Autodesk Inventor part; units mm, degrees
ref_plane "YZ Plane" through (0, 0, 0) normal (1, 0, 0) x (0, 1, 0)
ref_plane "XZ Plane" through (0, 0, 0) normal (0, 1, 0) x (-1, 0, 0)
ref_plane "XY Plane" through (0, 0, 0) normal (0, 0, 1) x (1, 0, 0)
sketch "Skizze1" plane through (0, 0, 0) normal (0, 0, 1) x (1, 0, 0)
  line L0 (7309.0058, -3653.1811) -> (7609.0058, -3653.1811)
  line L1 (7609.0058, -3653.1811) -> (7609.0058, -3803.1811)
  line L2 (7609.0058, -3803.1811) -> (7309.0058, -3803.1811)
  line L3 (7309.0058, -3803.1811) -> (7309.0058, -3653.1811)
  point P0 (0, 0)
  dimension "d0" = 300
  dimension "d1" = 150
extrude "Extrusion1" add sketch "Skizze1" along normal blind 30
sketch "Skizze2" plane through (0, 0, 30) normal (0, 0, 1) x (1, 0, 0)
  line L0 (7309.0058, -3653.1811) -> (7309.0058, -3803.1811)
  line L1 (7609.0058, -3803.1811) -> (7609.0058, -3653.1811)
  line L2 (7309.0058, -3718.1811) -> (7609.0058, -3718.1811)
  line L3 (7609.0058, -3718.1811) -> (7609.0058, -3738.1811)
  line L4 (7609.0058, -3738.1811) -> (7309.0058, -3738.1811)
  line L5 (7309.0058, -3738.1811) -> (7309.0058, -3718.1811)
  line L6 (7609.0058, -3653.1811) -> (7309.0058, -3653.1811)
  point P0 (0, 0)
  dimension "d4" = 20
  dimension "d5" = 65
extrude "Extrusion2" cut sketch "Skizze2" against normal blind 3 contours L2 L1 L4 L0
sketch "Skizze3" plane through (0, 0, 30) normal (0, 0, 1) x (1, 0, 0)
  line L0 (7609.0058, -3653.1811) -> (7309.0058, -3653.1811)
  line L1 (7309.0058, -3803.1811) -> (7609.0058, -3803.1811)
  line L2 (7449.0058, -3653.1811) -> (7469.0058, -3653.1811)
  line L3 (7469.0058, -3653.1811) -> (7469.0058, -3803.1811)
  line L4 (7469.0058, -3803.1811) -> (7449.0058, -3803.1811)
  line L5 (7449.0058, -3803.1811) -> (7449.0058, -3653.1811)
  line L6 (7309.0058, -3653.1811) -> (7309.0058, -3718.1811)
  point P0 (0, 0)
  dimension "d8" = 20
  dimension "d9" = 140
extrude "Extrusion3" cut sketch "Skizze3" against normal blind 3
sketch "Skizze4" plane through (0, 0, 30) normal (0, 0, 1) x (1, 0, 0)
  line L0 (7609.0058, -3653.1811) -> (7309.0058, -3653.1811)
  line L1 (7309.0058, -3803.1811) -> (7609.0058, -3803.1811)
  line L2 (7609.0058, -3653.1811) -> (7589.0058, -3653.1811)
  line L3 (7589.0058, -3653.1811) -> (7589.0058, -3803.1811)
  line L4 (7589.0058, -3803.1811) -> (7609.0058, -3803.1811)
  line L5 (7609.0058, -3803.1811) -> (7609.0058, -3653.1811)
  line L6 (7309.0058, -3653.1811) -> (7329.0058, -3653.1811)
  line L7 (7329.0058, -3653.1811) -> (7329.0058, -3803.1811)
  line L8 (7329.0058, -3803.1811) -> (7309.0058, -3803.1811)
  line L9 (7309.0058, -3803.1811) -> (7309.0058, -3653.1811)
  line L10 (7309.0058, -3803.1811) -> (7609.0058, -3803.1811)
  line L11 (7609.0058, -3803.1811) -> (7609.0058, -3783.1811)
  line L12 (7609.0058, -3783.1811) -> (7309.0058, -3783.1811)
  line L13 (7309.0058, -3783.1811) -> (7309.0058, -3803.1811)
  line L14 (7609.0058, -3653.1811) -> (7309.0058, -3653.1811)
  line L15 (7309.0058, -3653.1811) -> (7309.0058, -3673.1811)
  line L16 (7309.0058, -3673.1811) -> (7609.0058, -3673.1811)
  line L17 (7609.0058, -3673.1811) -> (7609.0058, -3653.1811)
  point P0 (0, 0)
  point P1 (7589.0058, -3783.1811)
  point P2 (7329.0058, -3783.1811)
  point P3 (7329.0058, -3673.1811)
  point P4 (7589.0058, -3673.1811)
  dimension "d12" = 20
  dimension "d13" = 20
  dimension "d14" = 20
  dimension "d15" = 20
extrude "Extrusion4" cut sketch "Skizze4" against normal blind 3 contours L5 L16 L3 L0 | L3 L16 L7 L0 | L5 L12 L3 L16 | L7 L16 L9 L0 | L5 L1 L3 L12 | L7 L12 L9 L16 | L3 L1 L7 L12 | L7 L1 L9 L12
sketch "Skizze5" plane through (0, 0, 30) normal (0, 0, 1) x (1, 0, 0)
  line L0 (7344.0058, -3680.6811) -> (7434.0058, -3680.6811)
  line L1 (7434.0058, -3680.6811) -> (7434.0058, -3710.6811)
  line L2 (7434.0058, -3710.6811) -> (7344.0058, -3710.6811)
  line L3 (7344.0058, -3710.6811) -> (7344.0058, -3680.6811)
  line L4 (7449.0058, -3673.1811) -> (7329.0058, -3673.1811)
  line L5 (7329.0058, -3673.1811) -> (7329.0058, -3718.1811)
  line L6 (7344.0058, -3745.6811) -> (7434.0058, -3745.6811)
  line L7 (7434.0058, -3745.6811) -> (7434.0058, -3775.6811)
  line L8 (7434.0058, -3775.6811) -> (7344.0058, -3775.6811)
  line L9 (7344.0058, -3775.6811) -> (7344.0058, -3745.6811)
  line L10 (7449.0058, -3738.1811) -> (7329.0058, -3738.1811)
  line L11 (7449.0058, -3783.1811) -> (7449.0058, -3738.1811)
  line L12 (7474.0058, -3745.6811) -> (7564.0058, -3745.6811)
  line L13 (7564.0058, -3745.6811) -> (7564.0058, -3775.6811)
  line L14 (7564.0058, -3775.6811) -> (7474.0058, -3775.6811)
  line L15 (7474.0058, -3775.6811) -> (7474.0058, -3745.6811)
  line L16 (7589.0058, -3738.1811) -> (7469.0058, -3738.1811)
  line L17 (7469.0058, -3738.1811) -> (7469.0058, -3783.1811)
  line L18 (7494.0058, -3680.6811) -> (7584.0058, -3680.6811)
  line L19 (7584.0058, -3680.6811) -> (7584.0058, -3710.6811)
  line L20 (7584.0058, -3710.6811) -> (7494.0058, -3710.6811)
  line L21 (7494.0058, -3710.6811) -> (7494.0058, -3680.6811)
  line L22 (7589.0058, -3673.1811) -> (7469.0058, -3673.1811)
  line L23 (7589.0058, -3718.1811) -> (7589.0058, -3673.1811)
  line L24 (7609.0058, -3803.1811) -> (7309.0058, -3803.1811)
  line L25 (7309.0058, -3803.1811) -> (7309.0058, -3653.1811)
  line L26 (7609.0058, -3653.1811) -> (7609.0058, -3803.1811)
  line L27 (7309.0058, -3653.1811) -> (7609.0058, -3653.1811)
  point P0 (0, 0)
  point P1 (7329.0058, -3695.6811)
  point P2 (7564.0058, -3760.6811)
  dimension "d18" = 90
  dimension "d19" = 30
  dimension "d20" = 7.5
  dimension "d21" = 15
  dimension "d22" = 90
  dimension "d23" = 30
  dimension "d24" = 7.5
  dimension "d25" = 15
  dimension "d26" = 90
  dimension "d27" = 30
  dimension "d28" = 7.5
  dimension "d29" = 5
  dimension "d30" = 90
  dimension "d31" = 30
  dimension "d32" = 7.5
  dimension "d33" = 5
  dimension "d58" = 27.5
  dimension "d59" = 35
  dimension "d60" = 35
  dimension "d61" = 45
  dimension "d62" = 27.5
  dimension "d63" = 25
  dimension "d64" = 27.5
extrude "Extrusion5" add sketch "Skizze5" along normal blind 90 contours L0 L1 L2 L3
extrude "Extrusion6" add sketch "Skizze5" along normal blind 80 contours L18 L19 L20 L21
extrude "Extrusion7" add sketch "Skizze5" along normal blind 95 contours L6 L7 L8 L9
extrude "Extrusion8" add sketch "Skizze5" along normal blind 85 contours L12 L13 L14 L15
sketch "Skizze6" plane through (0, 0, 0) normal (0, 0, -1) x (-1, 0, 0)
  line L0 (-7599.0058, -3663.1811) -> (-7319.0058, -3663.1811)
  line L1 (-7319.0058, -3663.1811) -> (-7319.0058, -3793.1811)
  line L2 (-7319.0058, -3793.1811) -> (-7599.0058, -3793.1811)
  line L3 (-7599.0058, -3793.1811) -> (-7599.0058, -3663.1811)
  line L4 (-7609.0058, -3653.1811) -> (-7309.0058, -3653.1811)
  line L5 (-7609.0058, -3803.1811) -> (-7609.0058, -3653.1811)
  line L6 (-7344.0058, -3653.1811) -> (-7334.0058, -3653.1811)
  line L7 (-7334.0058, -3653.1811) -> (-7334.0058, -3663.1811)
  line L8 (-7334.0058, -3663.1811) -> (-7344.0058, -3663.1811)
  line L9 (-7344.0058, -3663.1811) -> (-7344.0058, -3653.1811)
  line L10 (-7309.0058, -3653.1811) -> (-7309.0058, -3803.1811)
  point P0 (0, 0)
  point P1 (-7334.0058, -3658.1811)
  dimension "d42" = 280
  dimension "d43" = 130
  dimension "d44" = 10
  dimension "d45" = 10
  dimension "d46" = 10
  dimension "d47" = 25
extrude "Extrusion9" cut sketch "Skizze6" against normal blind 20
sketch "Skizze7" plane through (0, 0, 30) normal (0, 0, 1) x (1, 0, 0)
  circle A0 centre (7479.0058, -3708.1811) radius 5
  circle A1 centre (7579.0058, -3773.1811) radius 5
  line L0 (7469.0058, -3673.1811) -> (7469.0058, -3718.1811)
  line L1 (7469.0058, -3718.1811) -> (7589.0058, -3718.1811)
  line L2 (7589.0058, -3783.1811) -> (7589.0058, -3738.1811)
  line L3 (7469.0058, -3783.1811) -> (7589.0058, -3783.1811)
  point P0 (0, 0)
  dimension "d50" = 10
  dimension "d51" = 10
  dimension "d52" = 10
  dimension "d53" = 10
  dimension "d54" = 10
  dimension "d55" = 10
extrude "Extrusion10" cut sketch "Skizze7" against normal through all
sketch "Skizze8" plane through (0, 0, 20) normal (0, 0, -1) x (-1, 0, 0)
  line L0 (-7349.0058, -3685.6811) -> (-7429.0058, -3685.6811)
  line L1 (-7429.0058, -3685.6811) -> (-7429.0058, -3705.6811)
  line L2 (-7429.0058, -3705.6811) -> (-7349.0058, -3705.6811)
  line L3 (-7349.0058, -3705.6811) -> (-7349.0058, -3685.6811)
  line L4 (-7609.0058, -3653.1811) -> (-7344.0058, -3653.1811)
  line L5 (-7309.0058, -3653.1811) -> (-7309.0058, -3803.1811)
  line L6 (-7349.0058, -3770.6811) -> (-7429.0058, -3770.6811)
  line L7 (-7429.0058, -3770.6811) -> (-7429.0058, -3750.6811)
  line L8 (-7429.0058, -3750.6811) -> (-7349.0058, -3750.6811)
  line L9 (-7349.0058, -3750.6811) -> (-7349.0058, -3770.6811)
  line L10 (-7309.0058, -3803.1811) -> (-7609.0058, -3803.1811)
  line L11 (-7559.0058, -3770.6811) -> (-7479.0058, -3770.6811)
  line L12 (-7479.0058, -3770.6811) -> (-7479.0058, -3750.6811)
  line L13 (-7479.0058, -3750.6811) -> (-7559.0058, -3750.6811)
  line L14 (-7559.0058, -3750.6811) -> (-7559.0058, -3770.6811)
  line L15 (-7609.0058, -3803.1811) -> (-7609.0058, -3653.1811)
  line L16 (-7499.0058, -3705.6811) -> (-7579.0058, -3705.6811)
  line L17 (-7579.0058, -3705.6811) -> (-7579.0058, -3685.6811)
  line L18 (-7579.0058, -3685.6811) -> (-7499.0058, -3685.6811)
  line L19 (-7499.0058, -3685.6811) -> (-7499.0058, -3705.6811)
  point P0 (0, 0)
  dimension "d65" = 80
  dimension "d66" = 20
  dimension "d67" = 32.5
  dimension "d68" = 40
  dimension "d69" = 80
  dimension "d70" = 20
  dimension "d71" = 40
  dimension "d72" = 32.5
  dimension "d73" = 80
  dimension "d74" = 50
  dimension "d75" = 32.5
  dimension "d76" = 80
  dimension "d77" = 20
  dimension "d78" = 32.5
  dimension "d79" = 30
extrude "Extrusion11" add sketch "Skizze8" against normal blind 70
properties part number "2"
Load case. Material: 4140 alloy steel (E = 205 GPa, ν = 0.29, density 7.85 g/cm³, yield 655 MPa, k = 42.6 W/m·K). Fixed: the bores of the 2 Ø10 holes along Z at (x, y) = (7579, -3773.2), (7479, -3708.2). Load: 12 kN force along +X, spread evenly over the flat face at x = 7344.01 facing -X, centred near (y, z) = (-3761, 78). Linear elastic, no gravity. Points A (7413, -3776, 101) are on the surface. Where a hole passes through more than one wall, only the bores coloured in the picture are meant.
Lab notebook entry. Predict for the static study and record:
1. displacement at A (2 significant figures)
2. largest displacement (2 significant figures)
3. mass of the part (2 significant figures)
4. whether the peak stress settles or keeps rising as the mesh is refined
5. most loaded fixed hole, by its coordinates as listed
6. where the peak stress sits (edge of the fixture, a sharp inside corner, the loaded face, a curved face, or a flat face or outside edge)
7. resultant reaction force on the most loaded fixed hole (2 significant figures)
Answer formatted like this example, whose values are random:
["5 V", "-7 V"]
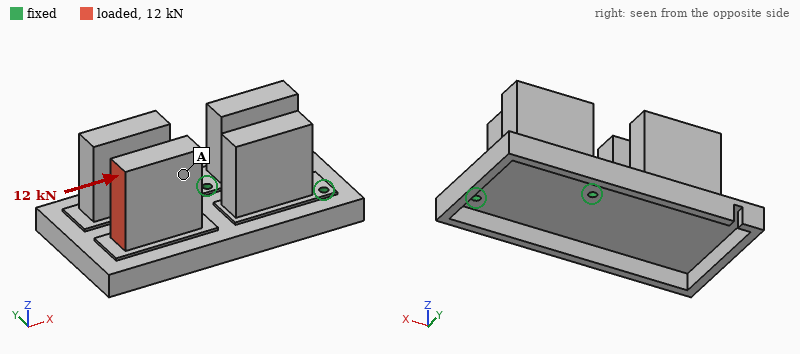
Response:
["0.76 mm", "1.3 mm", "12 kg", "keeps rising", "(7479, -3708.2)", "edge of the fixture", "9.6 kN"]
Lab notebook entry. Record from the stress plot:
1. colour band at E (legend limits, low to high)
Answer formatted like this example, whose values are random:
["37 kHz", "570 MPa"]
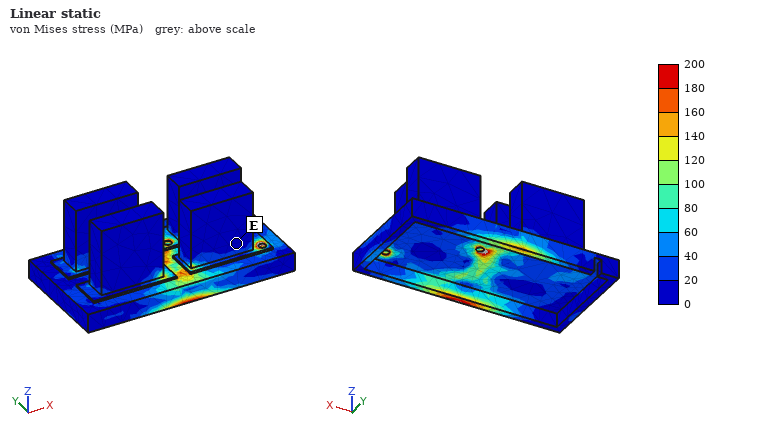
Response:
["0 to 20 MPa"]
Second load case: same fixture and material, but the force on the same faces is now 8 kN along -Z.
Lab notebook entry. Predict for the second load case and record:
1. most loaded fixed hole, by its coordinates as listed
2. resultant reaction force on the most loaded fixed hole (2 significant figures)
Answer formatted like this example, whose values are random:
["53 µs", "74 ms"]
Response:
["(7479, -3708.2)", "14 kN"]
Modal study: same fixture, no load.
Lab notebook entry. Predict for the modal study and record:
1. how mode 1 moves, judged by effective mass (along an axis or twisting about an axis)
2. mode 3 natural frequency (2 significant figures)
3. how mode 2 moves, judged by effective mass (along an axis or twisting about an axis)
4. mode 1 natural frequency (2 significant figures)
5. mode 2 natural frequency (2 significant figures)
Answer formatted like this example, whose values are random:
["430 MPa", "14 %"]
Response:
["along Z", "580 Hz", "along Y", "180 Hz", "340 Hz"]
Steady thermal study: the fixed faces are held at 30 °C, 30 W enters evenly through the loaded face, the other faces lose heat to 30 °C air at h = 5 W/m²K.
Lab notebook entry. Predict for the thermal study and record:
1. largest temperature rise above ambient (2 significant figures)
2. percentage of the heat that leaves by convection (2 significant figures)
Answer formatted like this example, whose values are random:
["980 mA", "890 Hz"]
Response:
["49 K", "54 %"]
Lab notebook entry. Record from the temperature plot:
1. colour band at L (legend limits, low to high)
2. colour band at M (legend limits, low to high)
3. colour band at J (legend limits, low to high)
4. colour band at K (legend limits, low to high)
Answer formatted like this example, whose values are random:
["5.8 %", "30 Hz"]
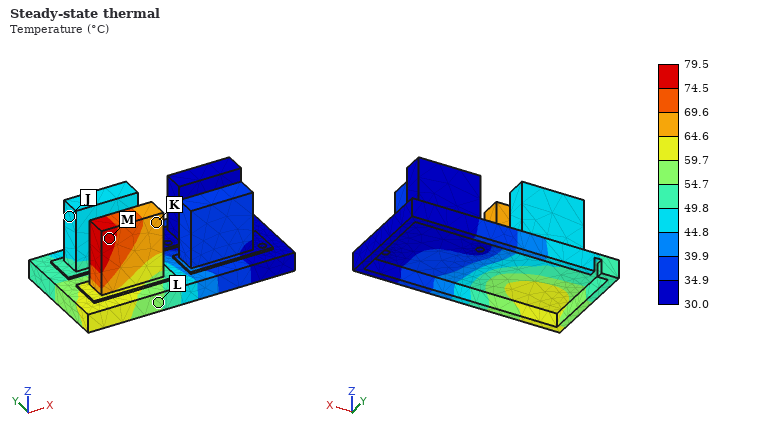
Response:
["54.7 to 59.7 °C", "74.5 to 79.5 °C", "44.8 to 49.8 °C", "64.6 to 69.6 °C"]
